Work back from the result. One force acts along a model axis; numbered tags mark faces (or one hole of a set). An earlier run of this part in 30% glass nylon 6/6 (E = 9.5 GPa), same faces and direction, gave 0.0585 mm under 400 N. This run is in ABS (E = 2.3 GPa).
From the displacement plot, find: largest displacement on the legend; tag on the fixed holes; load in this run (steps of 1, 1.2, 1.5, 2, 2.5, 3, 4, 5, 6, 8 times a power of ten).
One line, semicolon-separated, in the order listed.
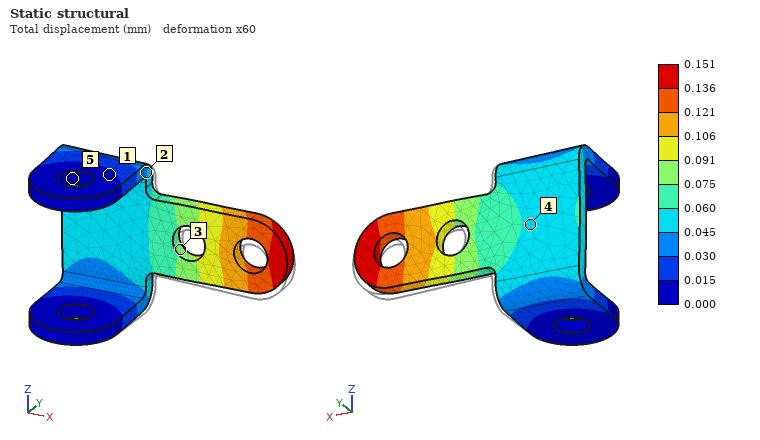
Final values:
0.151 mm; 5; 250 N
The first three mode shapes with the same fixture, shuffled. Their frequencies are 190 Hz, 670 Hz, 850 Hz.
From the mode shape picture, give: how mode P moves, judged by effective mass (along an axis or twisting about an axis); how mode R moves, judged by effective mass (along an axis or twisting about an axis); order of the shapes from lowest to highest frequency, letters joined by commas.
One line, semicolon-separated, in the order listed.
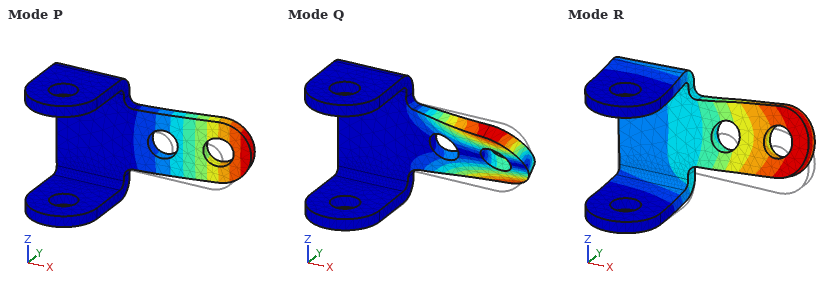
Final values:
along Y; along Z; P, R, Q
